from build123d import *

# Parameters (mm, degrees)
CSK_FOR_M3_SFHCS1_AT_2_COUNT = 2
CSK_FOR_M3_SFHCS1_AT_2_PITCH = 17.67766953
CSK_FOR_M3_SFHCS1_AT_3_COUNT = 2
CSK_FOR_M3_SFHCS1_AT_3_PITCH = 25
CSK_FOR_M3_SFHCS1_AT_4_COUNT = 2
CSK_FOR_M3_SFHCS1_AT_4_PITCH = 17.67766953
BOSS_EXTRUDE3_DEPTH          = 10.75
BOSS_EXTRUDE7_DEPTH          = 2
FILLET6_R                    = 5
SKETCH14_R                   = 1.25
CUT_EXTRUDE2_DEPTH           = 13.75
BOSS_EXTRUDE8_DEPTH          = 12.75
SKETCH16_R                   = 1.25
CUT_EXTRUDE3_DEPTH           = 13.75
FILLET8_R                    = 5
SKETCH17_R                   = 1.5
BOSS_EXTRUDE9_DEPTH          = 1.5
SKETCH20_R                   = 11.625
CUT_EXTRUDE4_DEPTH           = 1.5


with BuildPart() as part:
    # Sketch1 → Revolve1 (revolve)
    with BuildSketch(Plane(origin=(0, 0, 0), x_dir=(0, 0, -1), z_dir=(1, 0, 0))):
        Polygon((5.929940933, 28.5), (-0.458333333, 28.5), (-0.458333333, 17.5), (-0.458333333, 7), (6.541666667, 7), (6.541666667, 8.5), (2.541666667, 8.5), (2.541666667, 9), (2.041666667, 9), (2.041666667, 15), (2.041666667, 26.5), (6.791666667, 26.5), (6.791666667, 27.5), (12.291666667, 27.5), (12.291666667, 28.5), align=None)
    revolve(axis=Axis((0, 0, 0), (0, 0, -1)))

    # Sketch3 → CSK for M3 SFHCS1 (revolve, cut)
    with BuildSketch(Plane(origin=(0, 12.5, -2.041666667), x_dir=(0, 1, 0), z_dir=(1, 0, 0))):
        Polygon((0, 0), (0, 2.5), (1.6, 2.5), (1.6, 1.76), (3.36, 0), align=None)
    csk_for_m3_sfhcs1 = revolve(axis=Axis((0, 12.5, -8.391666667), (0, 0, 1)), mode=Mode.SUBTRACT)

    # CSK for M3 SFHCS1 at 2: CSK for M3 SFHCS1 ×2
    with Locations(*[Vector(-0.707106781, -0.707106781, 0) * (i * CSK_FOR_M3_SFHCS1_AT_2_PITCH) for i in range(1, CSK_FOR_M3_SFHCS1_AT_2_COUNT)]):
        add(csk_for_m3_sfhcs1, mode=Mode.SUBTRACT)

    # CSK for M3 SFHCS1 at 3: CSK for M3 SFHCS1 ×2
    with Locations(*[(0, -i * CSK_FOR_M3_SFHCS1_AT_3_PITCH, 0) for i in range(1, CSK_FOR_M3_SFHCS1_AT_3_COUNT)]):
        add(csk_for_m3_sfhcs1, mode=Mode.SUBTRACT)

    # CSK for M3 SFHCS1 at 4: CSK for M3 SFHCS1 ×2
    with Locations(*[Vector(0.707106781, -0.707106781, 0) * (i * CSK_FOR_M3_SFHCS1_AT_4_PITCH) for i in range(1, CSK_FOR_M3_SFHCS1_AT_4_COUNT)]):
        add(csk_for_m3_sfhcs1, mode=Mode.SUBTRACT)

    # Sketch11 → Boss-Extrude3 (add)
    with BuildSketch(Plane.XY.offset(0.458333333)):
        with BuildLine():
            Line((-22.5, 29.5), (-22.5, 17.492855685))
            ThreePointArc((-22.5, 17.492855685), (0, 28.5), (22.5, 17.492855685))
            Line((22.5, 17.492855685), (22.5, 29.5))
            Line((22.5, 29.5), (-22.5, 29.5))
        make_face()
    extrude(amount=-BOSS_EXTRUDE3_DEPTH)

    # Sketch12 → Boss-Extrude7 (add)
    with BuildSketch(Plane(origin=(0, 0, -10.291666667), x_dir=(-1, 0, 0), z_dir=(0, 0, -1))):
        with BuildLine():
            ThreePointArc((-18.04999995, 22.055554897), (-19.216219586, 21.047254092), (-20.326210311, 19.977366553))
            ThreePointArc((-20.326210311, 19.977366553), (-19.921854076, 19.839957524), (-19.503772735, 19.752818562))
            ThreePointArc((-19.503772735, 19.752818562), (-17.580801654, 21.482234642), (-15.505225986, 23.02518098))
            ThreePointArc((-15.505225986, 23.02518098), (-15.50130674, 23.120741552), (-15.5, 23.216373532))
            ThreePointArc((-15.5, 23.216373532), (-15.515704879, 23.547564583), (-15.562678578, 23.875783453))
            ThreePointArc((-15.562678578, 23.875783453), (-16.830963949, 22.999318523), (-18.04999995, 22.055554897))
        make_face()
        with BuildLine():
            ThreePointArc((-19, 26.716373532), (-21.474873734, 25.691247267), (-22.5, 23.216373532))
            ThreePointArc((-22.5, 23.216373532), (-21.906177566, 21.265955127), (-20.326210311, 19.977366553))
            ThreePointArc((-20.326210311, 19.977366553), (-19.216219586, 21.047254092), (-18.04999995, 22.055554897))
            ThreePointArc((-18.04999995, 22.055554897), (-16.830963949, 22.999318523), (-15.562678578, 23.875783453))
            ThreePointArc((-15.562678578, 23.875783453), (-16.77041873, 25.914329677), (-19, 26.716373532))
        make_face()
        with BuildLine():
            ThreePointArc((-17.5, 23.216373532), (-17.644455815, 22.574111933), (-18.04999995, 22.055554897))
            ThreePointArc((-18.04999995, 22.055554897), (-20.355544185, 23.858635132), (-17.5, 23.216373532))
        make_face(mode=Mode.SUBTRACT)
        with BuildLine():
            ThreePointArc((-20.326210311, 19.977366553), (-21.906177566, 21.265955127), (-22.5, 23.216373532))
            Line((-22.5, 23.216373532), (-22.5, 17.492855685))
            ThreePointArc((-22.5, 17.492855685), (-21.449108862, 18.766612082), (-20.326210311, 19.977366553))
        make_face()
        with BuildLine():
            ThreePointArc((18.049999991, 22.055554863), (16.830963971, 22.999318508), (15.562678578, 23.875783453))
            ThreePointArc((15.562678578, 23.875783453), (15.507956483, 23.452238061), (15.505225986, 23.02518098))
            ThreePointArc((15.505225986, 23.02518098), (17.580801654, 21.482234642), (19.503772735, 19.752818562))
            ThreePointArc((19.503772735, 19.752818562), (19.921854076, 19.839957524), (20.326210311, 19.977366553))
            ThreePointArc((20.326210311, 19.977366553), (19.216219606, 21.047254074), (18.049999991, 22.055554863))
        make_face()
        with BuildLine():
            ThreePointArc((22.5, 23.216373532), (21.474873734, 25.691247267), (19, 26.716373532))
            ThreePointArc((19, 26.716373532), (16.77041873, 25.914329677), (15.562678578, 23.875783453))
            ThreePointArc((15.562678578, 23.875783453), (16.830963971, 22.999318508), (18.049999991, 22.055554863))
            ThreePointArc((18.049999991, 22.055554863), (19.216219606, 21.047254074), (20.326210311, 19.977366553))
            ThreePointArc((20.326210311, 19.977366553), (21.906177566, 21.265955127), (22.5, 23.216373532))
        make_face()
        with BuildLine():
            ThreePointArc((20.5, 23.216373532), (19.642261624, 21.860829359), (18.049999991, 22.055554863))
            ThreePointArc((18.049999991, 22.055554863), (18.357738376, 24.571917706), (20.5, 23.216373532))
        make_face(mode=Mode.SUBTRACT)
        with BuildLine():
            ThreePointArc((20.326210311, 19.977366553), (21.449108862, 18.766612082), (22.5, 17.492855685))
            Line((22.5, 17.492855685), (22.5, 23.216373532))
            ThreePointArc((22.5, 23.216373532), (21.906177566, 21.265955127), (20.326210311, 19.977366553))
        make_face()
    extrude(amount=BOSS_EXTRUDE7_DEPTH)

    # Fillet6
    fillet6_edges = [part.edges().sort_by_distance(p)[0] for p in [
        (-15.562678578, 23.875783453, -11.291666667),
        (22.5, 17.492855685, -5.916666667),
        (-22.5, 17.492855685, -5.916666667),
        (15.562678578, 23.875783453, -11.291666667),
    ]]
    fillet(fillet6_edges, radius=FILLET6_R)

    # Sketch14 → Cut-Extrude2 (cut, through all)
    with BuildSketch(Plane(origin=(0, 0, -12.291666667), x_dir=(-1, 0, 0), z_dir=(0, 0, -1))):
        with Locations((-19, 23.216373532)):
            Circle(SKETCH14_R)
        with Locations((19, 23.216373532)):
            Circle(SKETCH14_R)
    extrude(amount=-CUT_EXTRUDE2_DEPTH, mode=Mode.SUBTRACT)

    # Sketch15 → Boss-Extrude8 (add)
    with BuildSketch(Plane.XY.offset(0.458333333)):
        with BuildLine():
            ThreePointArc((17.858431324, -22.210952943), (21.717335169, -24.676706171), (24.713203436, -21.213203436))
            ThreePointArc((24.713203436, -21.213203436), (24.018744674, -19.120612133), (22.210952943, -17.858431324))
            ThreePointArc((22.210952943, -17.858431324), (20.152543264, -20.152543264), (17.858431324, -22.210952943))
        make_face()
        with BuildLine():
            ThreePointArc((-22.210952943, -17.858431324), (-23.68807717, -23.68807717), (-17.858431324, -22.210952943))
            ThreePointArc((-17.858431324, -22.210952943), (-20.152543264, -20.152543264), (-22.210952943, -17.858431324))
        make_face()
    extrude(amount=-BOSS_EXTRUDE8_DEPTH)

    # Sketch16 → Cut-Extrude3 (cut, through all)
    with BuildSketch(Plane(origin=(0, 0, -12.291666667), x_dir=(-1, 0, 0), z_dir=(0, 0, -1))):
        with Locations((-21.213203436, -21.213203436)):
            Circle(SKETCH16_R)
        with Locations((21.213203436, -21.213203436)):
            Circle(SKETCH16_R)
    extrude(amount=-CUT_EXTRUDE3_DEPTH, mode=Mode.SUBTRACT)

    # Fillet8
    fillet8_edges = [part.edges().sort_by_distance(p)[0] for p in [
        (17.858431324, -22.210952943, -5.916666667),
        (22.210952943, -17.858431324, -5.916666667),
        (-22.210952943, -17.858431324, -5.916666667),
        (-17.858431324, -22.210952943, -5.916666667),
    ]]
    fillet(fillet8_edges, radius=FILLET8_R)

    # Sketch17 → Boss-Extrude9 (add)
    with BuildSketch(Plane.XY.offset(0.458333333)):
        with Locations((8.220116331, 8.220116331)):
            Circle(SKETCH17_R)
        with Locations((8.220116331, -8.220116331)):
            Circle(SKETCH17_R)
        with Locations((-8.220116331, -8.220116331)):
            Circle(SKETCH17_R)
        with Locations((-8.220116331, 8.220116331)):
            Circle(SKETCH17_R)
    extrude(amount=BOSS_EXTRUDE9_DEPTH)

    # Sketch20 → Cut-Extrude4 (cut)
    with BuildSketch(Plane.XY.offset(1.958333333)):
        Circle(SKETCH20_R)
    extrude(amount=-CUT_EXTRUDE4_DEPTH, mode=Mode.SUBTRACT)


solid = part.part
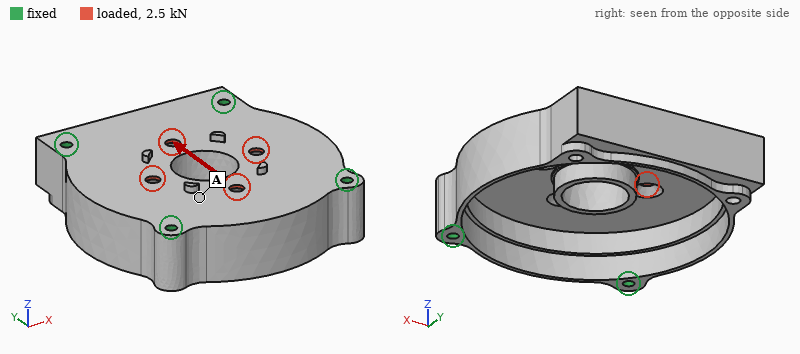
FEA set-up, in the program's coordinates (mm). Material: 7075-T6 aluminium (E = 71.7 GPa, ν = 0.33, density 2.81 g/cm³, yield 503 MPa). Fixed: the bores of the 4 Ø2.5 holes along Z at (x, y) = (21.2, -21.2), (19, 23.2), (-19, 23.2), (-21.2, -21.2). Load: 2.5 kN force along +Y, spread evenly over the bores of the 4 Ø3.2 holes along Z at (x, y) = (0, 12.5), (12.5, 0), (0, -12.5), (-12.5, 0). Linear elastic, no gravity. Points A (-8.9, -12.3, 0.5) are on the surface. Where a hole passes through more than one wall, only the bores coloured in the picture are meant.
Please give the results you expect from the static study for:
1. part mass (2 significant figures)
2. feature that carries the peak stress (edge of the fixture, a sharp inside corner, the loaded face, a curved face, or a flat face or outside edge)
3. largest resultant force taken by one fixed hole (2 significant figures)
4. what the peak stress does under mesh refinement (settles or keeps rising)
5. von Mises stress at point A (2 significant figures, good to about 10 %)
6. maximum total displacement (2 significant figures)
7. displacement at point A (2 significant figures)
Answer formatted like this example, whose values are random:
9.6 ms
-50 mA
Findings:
33 g
a sharp inside corner
680 N
keeps rising
13 MPa
11 µm
5.5 µm
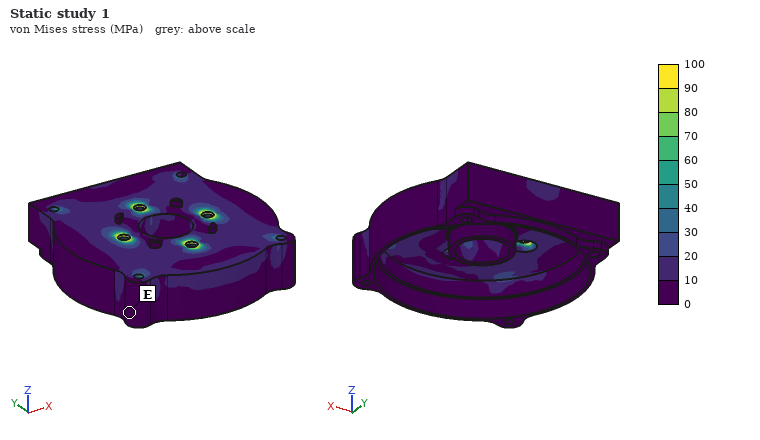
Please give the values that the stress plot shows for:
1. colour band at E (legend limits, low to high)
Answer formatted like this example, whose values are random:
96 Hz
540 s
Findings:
0 to 10 MPa
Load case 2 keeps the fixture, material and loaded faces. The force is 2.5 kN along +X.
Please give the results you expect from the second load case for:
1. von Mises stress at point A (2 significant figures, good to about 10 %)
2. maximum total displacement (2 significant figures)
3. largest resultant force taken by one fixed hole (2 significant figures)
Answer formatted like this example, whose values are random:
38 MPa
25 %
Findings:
17 MPa
11 µm
660 N
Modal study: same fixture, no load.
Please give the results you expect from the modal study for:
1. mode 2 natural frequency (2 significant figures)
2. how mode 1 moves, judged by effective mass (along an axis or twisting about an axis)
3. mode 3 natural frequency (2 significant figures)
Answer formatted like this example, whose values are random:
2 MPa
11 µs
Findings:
13 kHz
along Z
13 kHz
